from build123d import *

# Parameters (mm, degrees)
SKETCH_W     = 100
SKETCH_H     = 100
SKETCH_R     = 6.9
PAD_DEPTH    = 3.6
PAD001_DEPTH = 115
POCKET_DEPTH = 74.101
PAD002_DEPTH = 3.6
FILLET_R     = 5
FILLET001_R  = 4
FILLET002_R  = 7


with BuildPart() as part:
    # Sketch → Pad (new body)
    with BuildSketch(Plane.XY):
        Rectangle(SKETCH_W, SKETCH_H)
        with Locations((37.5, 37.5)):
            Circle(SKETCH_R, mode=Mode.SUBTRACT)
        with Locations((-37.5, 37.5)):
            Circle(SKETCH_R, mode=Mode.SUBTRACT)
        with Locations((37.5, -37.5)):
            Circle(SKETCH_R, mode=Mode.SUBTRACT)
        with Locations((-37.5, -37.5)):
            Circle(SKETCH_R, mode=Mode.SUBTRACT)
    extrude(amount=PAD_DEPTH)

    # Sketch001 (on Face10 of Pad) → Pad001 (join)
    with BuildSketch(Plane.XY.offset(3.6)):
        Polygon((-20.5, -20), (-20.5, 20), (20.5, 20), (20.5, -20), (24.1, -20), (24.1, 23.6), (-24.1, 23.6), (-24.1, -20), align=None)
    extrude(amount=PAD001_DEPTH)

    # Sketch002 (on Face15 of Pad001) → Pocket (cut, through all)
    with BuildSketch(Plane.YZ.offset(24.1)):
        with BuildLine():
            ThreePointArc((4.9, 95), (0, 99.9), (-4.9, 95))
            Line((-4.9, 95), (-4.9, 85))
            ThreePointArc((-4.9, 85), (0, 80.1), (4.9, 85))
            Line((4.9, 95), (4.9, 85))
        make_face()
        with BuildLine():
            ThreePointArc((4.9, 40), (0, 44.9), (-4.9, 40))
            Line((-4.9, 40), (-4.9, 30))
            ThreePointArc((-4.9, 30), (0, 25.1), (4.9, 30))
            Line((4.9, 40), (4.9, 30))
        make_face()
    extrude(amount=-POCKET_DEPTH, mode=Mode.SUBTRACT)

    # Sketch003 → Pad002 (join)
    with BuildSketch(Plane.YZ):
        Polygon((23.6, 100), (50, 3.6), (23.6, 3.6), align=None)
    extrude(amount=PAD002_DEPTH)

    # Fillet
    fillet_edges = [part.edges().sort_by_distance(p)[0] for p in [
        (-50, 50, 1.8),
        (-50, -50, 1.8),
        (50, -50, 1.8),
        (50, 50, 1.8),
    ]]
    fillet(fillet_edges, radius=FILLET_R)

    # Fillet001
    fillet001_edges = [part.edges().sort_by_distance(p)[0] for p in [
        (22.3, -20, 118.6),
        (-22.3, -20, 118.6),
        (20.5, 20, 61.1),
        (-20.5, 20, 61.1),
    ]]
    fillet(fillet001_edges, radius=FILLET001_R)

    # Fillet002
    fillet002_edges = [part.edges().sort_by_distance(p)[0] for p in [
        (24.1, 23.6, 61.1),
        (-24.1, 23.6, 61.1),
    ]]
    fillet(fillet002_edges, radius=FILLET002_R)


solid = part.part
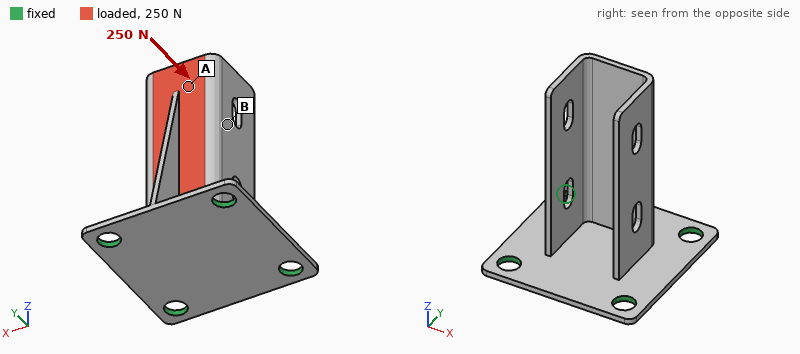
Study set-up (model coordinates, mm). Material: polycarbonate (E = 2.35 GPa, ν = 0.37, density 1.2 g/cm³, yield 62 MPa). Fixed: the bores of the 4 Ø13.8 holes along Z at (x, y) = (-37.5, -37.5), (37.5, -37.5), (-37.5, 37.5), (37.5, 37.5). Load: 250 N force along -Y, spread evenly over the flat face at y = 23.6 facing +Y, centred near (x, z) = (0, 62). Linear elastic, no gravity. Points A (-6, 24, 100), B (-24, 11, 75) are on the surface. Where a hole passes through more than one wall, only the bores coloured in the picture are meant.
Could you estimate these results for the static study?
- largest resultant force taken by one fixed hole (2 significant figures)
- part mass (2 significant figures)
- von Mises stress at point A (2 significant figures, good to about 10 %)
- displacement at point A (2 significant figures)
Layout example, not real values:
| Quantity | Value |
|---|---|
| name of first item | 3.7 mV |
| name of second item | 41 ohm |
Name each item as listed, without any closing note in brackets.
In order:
| Quantity | Value |
|---|---|
| largest resultant force taken by one fixed hole | 140 N |
| part mass | 100 g |
| von Mises stress at point A | 4.4 MPa |
| displacement at point A | 1.8 mm |
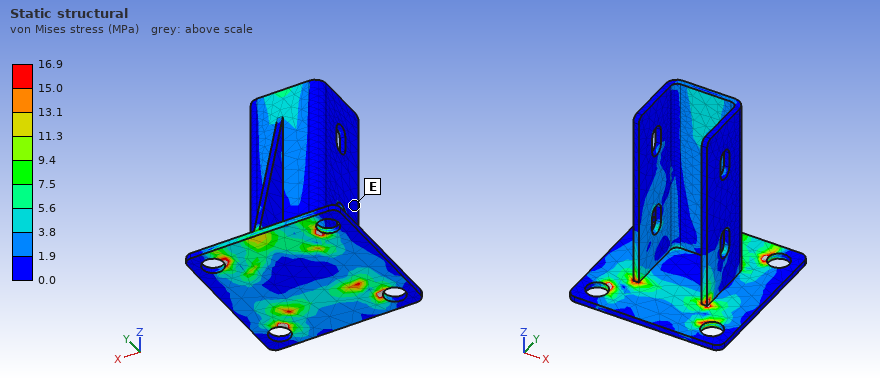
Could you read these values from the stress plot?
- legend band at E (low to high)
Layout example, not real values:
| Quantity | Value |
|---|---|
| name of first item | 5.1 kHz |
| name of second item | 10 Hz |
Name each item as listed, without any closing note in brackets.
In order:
| Quantity | Value |
|---|---|
| legend band at E | 0.0 to 1.9 MPa |
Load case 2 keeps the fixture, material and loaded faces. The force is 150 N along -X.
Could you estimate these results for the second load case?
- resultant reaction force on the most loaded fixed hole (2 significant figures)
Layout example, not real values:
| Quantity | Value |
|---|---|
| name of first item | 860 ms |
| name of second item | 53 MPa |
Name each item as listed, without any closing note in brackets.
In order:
| Quantity | Value |
|---|---|
| resultant reaction force on the most loaded fixed hole | 130 N |
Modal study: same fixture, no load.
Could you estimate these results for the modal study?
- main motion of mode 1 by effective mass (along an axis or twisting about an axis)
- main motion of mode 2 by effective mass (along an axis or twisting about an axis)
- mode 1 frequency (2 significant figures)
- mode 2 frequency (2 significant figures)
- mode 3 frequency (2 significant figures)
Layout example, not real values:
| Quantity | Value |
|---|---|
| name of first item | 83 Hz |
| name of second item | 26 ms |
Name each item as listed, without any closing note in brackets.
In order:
| Quantity | Value |
|---|---|
| main motion of mode 1 by effective mass | along X |
| main motion of mode 2 by effective mass | along Y |
| mode 1 frequency | 180 Hz |
| mode 2 frequency | 280 Hz |
| mode 3 frequency | 350 Hz |
